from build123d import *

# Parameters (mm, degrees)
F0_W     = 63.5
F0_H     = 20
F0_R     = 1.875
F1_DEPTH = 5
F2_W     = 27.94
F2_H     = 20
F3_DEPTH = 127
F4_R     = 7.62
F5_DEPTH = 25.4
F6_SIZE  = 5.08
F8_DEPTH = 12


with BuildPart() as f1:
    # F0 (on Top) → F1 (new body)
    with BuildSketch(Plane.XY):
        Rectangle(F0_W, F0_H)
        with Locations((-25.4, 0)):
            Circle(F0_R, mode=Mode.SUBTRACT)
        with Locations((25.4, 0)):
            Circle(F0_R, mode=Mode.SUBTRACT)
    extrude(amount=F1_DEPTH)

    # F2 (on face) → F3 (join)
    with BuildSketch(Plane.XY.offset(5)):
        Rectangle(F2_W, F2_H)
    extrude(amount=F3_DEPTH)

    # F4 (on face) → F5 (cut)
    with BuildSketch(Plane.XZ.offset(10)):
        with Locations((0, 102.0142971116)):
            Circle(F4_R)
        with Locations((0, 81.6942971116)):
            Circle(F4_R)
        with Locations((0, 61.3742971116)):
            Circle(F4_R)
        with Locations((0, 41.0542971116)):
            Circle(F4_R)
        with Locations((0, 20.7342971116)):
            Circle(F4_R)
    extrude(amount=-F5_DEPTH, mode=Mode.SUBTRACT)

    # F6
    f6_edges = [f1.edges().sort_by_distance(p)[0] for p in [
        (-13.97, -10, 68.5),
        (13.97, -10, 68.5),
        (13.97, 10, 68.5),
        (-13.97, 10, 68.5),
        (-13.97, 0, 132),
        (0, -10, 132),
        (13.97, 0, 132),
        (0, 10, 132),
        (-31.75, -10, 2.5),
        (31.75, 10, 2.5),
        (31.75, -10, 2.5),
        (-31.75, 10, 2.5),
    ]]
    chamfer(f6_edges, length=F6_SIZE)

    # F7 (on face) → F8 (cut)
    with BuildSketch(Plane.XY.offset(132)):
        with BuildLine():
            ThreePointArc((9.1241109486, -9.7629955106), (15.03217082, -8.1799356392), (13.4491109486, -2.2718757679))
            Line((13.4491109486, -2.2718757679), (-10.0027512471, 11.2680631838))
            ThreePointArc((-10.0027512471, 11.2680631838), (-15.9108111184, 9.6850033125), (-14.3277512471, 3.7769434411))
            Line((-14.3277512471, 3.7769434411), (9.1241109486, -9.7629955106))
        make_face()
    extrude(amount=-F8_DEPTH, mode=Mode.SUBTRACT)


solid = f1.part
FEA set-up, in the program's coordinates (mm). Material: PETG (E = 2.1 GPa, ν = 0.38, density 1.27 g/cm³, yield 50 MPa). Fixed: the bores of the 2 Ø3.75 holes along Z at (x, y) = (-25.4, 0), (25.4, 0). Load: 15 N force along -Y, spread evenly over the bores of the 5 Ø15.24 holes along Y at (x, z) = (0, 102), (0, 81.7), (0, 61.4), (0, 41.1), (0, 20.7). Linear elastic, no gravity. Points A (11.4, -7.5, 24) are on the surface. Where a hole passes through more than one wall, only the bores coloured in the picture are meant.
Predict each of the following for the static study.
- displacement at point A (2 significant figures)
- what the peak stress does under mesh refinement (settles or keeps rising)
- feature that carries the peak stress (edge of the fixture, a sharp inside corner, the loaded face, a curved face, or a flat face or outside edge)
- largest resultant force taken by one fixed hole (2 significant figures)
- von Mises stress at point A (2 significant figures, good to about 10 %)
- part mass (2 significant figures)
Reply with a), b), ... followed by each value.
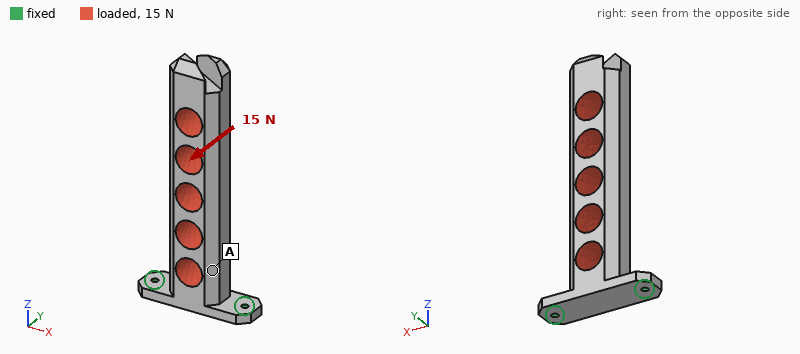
a) 0.23 mm
b) keeps rising
c) edge of the fixture
d) 7.5 N
e) 0.73 MPa
f) 62 g
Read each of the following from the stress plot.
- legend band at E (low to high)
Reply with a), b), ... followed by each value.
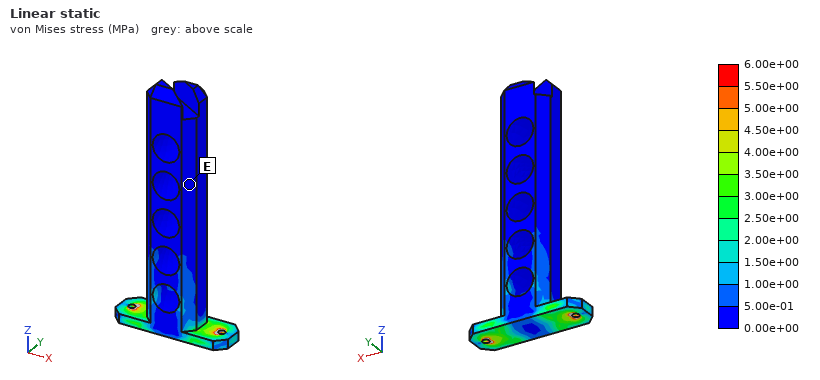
a) 0.00e+00 to 5.00e-01 MPa
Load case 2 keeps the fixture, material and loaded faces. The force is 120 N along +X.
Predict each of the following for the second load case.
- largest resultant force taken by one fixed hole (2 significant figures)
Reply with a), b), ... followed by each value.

a) 190 N
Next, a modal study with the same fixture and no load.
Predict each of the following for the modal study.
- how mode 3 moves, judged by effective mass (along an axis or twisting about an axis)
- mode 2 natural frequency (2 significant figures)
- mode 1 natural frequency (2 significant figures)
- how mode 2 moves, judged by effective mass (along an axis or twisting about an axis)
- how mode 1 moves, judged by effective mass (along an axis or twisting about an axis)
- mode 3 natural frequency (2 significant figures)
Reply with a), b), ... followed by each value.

a) along Y
b) 220 Hz
c) 81 Hz
d) along X
e) along Y
f) 810 Hz
